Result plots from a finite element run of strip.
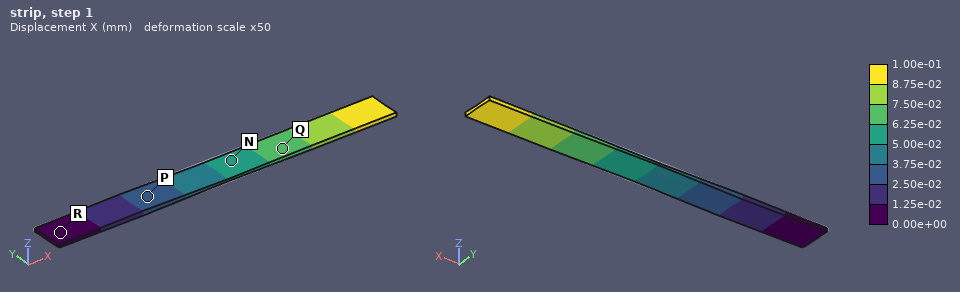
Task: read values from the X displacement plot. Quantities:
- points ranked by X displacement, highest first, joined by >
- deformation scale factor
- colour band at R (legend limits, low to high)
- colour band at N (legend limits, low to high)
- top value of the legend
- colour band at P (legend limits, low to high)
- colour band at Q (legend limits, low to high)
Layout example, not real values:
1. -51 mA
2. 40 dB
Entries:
1. Q > N > P > R
2. 50
3. 0.00e+00 to 1.25e-02 mm
4. 5.00e-02 to 6.25e-02 mm
5. 1.00e-01 mm
6. 2.50e-02 to 3.75e-02 mm
7. 6.25e-02 to 7.50e-02 mm
